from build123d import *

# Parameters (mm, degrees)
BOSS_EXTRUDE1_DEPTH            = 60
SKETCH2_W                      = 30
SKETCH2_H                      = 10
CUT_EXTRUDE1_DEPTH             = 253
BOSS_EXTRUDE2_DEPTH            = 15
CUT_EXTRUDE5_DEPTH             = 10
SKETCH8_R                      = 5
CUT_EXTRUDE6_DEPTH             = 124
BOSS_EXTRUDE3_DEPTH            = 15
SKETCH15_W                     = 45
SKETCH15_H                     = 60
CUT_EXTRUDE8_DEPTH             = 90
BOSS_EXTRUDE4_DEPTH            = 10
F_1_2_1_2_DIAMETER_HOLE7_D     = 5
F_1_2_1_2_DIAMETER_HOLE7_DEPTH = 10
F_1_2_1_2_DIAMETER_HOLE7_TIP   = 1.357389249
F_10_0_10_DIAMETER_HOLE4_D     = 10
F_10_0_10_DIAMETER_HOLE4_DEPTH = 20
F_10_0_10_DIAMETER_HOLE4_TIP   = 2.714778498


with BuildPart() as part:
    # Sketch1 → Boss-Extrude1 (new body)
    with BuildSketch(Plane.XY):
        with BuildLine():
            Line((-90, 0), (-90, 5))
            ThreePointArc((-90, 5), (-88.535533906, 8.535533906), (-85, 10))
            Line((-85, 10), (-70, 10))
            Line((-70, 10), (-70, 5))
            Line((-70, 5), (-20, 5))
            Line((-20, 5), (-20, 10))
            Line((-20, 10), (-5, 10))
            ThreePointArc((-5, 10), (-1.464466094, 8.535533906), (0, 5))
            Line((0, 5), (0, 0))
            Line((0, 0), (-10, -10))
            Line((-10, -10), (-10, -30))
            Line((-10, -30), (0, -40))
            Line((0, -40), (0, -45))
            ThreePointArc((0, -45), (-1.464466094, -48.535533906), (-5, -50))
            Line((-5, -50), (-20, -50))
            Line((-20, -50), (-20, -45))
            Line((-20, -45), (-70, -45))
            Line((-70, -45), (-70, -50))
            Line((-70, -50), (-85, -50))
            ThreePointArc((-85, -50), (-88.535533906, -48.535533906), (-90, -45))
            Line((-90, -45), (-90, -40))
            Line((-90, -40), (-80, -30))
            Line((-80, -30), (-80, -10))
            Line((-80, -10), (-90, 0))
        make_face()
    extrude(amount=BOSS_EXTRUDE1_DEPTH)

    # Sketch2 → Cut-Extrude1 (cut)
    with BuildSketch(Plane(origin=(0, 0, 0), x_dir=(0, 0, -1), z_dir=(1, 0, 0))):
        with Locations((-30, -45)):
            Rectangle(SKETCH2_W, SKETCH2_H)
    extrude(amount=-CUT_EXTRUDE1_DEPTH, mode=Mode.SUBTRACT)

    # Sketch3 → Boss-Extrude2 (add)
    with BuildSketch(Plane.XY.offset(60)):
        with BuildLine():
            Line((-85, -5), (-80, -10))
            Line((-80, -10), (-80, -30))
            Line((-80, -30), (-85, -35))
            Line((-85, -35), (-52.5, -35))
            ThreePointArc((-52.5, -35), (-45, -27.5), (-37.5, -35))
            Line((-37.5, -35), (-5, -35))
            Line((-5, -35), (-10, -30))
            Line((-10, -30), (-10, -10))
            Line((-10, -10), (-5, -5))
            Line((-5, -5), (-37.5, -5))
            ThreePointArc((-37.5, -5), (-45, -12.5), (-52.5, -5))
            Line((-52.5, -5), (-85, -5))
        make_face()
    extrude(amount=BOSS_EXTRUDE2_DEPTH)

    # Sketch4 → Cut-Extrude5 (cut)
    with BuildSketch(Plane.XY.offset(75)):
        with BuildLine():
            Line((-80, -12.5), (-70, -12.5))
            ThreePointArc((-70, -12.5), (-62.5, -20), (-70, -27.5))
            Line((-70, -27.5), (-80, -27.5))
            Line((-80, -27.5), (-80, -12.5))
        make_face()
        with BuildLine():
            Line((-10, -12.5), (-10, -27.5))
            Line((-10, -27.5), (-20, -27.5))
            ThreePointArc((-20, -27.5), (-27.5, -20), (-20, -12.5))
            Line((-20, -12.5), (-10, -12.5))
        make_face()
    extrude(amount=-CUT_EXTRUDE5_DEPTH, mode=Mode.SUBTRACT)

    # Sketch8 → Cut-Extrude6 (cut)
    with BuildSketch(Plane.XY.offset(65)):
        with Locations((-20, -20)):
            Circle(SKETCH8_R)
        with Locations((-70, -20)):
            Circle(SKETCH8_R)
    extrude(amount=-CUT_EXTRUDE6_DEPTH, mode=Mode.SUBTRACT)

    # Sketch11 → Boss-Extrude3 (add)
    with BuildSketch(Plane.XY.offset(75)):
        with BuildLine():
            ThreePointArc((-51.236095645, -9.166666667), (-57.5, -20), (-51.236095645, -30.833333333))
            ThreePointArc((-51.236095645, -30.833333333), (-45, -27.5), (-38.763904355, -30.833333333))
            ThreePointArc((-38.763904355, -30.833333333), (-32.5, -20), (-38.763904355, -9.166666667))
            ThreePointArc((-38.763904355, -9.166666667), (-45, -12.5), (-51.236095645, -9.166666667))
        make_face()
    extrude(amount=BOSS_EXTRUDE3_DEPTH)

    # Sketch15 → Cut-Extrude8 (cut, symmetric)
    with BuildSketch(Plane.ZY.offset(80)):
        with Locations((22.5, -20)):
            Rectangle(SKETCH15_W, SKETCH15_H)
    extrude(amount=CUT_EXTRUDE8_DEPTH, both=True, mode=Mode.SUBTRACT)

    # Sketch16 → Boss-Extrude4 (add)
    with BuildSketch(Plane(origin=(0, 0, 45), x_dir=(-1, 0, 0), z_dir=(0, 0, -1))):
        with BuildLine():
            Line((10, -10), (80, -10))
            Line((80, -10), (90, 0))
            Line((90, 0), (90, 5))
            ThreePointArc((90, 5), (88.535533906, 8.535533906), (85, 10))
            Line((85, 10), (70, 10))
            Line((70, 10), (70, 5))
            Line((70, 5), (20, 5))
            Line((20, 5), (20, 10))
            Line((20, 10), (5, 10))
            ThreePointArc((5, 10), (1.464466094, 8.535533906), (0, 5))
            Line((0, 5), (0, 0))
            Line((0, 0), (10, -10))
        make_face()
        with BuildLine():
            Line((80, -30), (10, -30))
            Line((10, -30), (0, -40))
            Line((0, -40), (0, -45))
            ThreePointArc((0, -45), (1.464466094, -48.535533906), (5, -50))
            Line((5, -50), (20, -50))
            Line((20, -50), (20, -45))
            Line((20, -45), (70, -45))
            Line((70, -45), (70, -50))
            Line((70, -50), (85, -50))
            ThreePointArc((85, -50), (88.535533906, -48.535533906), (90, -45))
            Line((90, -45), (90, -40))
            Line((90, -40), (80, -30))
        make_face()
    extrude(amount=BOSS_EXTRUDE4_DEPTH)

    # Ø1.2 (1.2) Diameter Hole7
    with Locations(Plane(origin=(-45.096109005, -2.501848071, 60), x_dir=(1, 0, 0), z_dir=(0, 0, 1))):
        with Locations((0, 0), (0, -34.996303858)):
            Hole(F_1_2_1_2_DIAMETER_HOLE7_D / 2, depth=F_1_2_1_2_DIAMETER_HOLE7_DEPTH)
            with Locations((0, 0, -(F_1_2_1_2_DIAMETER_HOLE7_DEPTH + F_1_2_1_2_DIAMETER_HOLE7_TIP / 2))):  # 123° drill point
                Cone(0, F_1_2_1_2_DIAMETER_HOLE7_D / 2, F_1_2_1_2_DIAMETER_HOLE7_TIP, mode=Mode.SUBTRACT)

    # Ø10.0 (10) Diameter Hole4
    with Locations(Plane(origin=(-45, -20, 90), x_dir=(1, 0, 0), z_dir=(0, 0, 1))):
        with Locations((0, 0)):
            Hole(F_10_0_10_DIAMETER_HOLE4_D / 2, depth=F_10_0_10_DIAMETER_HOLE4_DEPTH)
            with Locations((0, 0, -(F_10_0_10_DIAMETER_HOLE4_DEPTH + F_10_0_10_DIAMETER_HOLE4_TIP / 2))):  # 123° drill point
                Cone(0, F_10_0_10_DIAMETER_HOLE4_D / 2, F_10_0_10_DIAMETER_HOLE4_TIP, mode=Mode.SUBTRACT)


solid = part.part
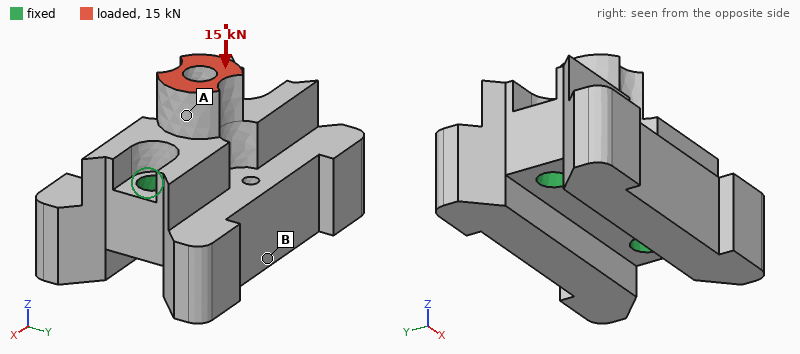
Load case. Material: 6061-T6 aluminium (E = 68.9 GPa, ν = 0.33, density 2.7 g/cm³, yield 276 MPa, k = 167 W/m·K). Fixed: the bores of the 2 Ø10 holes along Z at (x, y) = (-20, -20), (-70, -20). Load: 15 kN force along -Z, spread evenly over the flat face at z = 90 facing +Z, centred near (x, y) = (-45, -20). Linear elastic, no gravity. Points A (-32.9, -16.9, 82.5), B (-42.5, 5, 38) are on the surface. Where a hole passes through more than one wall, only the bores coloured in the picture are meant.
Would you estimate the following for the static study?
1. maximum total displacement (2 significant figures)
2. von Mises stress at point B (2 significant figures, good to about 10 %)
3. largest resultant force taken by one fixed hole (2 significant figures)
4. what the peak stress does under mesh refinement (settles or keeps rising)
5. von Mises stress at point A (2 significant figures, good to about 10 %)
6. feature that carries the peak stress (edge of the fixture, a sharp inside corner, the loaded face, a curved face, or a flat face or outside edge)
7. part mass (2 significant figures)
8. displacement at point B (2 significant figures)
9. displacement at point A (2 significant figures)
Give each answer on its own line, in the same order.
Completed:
22 µm
7.1 MPa
7.7 kN
keeps rising
48 MPa
edge of the fixture
320 g
5.8 µm
17 µm
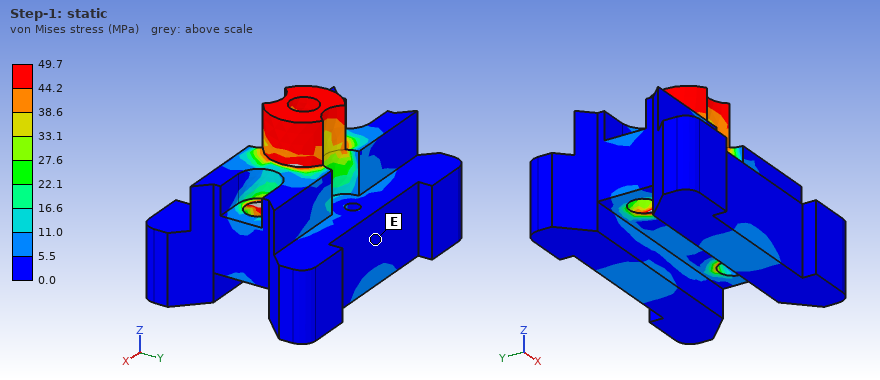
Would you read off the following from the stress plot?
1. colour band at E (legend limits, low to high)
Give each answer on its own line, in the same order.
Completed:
0.0 to 5.5 MPa
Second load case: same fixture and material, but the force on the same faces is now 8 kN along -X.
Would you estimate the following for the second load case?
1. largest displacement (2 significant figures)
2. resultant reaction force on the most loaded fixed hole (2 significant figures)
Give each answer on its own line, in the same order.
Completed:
62 µm
6.6 kN
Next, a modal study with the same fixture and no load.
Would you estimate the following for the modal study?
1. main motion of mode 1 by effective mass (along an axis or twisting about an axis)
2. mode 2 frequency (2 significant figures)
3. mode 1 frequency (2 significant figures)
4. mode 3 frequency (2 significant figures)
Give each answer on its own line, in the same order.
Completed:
twisting about X
12 kHz
9700 Hz
13 kHz
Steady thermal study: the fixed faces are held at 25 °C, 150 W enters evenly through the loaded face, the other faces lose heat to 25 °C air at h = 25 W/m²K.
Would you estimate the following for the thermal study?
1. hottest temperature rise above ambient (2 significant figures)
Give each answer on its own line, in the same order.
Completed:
66 K
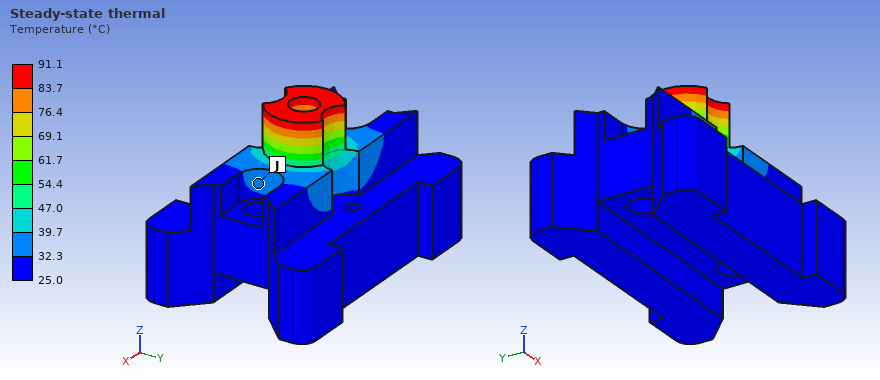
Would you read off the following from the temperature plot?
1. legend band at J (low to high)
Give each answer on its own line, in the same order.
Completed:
32.3 to 39.7 °C
